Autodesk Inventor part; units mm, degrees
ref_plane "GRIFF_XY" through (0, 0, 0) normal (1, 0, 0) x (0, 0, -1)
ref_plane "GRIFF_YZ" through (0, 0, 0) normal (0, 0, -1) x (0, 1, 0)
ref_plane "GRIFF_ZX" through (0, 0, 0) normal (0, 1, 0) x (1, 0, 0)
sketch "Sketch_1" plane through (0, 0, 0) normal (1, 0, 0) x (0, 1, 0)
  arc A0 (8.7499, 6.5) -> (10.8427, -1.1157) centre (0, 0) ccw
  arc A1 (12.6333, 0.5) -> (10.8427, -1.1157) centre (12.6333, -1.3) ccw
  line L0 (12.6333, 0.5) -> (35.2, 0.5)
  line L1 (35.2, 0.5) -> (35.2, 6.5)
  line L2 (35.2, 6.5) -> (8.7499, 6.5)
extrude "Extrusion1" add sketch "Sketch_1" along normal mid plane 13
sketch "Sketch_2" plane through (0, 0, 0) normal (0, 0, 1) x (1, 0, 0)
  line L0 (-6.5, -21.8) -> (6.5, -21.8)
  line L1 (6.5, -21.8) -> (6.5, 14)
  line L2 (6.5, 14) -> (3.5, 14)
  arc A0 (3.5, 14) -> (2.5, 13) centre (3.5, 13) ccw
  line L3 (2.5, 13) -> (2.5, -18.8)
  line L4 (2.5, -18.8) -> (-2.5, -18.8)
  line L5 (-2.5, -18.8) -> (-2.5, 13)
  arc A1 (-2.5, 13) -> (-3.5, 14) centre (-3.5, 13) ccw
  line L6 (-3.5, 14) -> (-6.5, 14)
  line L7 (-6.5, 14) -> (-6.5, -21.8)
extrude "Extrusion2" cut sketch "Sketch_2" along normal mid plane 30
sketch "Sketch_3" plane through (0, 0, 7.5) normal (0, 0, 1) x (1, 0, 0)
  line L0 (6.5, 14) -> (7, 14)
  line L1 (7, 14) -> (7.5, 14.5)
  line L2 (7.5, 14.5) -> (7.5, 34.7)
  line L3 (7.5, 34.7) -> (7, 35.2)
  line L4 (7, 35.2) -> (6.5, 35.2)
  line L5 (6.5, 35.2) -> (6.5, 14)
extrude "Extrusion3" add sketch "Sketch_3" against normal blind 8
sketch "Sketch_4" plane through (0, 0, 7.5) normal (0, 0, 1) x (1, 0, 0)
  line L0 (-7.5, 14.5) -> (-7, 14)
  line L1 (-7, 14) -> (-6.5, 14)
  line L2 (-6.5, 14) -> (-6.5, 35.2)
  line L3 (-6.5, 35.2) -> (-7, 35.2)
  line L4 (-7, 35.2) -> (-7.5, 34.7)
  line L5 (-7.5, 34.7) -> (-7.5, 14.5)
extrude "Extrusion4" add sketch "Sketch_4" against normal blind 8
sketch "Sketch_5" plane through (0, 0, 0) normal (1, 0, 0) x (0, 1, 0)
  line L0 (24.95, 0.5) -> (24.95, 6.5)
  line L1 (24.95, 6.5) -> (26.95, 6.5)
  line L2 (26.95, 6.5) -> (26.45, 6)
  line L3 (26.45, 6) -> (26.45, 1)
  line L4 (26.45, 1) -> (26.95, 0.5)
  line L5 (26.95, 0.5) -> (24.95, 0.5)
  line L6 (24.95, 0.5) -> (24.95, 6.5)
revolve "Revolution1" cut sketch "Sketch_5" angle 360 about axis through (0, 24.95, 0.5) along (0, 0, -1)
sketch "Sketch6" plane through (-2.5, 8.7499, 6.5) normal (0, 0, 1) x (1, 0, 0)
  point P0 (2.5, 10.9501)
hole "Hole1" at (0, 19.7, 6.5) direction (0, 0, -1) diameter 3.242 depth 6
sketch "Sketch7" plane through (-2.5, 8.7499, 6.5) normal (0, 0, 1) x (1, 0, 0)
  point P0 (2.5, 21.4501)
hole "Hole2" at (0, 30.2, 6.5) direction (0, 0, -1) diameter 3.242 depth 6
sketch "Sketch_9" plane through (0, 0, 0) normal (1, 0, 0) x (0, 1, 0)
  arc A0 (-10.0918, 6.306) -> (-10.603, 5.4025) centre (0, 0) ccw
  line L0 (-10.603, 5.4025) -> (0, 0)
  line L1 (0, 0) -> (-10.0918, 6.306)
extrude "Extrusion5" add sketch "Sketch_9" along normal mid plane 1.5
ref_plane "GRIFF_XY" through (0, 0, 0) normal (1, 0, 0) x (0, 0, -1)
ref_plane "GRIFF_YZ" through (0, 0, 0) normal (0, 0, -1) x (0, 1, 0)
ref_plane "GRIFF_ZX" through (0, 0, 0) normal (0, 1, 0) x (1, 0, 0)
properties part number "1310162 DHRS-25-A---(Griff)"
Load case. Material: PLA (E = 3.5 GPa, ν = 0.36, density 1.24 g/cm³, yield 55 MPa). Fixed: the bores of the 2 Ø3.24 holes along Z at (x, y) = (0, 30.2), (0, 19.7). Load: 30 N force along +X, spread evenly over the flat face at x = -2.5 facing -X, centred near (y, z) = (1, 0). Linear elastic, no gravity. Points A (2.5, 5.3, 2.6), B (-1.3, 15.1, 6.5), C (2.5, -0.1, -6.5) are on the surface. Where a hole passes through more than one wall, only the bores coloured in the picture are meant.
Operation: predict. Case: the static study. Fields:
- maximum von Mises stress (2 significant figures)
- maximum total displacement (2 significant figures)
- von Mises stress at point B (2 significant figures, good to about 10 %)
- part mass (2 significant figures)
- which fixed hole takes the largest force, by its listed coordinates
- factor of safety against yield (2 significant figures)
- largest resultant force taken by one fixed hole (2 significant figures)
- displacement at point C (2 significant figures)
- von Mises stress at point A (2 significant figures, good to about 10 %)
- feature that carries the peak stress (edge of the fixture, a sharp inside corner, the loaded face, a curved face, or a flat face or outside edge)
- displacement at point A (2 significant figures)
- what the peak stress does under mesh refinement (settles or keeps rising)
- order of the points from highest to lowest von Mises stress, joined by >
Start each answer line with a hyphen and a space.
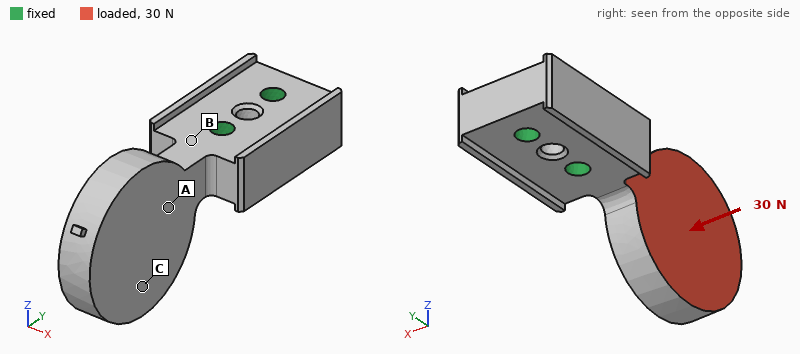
- 27 MPa
- 0.32 mm
- 6.4 MPa
- 4.8 g
- (0, 19.7)
- 2.1
- 61 N
- 0.20 mm
- 3.6 MPa
- the loaded face
- 0.094 mm
- settles
- B > A > C
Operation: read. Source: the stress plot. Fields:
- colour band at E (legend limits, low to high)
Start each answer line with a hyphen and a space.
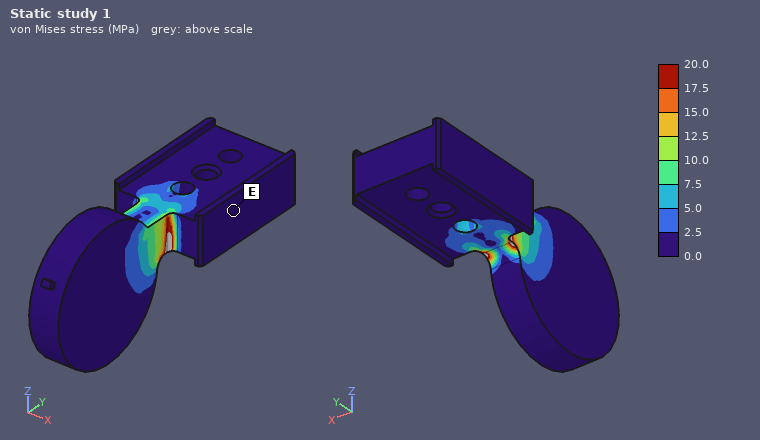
- 0.0 to 2.5 MPa
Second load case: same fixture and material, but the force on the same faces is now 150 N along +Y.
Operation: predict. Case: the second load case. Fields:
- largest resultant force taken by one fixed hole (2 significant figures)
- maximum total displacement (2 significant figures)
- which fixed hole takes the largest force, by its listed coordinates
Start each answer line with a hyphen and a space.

- 130 N
- 0.48 mm
- (0, 19.7)
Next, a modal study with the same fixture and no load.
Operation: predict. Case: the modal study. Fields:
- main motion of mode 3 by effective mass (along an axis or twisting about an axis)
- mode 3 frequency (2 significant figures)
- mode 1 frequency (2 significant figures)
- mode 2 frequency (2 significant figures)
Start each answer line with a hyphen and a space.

- twisting about Y
- 2700 Hz
- 1200 Hz
- 1300 Hz
